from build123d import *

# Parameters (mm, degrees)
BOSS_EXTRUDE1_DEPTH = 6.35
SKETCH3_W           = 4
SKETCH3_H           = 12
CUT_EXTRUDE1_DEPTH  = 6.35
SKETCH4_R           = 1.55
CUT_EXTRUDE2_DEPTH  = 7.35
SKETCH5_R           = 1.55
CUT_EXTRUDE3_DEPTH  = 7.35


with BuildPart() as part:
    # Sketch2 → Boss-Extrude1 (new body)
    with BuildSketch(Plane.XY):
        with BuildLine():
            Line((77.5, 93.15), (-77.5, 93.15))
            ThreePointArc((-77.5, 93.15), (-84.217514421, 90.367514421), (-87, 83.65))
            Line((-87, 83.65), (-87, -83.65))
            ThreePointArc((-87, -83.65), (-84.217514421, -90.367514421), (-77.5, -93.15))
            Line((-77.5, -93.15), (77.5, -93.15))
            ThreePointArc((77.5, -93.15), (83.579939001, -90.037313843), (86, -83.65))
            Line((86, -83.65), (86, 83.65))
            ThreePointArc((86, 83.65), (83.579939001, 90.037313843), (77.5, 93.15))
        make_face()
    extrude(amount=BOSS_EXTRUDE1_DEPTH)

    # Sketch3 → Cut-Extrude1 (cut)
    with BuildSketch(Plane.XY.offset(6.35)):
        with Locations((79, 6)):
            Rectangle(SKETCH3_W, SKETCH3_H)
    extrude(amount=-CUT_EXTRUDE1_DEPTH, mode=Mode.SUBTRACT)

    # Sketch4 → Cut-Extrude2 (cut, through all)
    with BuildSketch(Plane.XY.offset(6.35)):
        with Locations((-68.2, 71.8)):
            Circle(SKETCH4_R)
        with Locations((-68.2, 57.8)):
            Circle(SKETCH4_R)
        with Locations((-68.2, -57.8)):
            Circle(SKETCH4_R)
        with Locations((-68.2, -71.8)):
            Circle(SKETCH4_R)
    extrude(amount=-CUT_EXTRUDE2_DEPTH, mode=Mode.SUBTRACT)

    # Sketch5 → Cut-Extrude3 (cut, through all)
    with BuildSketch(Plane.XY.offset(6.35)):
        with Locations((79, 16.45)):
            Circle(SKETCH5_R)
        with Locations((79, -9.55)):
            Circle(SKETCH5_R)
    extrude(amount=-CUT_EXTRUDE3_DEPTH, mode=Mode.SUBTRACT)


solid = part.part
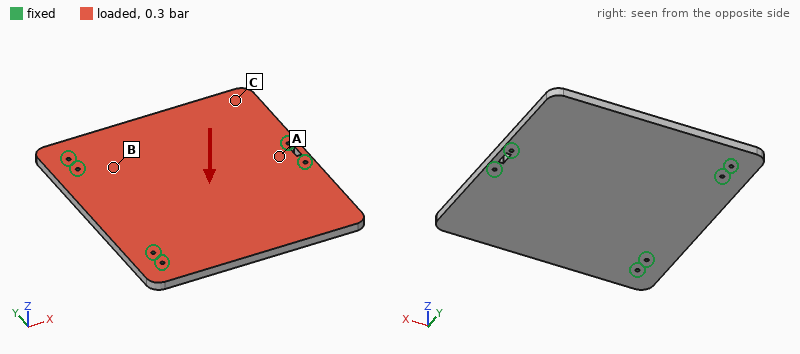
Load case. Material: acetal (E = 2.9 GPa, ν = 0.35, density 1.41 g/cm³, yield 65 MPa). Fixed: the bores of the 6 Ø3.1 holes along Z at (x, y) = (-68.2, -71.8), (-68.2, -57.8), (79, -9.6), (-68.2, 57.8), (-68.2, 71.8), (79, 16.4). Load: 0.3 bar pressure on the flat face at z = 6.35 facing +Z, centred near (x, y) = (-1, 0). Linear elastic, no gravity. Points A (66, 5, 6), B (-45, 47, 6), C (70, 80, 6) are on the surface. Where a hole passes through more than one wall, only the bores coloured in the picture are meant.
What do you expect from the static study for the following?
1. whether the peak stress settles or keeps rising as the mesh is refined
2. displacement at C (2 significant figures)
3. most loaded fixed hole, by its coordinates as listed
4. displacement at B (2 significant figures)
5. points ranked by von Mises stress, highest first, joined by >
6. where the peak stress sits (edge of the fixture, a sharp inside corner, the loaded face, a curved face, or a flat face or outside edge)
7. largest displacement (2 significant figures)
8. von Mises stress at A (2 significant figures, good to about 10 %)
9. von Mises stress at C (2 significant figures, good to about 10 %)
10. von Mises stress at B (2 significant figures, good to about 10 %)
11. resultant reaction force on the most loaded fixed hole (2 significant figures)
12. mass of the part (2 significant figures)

keeps rising
1.8 mm
(79, -9.6)
0.46 mm
A > B > C
edge of the fixture
2.9 mm
7.4 MPa
2.3 MPa
3.8 MPa
230 N
290 g
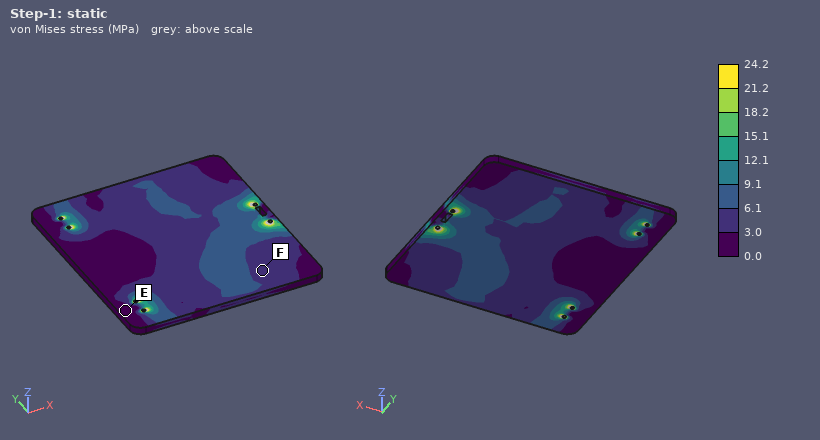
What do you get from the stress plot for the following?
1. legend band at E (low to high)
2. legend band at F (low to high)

0.0 to 3.0 MPa
3.0 to 6.1 MPa
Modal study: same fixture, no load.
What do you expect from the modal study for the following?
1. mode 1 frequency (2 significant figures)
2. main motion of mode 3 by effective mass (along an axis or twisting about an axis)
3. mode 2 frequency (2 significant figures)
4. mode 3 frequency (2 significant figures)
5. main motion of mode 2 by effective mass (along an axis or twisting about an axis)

220 Hz
along Z
240 Hz
380 Hz
along Z
